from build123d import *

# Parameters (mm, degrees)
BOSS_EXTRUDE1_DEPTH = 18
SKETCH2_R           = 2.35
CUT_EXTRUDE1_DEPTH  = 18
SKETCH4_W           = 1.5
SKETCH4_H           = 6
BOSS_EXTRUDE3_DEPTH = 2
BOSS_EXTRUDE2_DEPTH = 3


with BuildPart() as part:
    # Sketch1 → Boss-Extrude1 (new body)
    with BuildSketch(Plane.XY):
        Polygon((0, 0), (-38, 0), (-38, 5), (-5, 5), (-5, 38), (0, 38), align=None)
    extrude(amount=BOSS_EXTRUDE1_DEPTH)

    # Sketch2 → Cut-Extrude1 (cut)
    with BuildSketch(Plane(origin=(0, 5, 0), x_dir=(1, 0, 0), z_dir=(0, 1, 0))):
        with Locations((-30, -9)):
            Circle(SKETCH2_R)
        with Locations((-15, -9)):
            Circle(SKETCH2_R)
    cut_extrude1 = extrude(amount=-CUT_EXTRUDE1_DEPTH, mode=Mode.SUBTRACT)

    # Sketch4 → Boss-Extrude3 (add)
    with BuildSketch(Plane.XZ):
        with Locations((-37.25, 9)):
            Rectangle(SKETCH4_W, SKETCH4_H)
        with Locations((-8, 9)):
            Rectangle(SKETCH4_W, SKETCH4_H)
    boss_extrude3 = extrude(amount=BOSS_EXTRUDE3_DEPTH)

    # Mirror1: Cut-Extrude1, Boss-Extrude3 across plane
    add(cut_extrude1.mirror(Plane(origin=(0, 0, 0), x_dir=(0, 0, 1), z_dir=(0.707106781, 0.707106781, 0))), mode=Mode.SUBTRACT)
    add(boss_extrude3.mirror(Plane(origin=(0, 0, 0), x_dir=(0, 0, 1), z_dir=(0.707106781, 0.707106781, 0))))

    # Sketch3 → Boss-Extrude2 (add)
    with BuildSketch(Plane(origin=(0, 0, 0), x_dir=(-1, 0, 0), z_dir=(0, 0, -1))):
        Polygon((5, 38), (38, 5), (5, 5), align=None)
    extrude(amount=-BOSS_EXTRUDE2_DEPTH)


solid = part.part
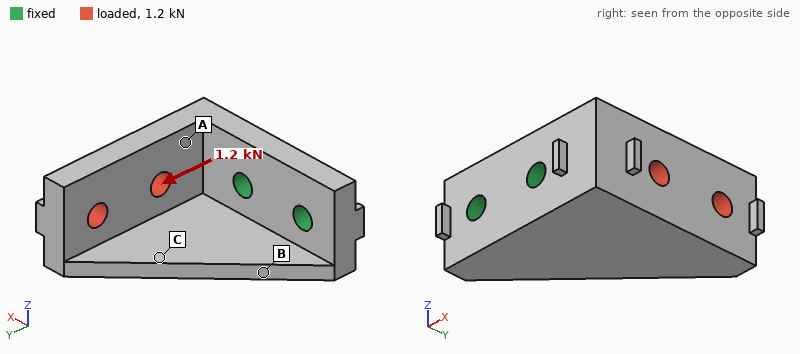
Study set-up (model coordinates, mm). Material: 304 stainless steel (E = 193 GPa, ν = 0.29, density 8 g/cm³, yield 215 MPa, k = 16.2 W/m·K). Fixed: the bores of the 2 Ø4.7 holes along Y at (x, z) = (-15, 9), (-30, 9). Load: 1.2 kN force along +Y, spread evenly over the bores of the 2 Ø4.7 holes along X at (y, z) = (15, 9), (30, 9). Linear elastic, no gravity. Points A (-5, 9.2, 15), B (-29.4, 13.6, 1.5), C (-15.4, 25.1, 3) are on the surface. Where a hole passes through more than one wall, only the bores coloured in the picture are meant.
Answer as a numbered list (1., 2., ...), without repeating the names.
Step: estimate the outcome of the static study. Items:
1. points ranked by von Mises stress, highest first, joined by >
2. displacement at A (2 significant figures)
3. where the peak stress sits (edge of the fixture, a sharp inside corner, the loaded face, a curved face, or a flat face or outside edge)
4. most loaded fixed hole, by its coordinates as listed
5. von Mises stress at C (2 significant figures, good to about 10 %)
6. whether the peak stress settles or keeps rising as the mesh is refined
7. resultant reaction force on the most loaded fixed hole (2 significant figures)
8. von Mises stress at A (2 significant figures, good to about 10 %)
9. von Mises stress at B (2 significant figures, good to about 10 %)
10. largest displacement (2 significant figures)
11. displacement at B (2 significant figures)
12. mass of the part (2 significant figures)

1. A > B > C
2. 11 µm
3. edge of the fixture
4. (-15, 9)
5. 11 MPa
6. keeps rising
7. 1.7 kN
8. 33 MPa
9. 26 MPa
10. 26 µm
11. 4.5 µm
12. 62 g
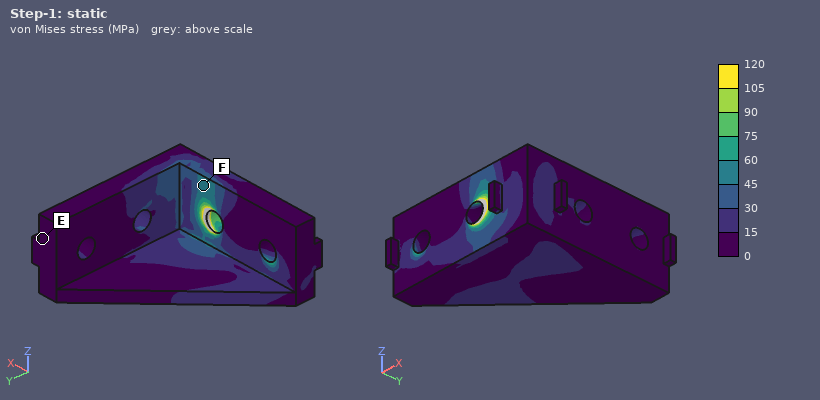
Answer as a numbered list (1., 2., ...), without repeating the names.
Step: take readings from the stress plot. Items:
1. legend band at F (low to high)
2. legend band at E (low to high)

1. 45 to 60 MPa
2. 0 to 15 MPa
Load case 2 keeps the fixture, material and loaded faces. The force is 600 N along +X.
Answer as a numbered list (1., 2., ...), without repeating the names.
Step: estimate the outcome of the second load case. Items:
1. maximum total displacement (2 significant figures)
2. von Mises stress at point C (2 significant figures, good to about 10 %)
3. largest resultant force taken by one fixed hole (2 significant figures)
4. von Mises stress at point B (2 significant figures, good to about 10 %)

1. 43 µm
2. 33 MPa
3. 620 N
4. 30 MPa
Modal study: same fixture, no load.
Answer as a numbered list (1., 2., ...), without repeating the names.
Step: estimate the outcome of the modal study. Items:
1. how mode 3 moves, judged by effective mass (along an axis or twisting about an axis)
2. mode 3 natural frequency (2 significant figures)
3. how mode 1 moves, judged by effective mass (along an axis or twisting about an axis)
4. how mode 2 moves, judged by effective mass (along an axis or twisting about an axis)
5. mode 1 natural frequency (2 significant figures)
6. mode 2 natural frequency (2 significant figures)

1. along Y
2. 10 kHz
3. along Z
4. along X
5. 3400 Hz
6. 5300 Hz
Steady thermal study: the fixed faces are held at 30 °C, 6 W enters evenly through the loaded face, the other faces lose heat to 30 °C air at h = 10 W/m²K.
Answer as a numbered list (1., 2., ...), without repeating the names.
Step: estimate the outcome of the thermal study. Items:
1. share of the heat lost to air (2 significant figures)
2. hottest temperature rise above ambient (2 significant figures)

1. 22 %
2. 74 K
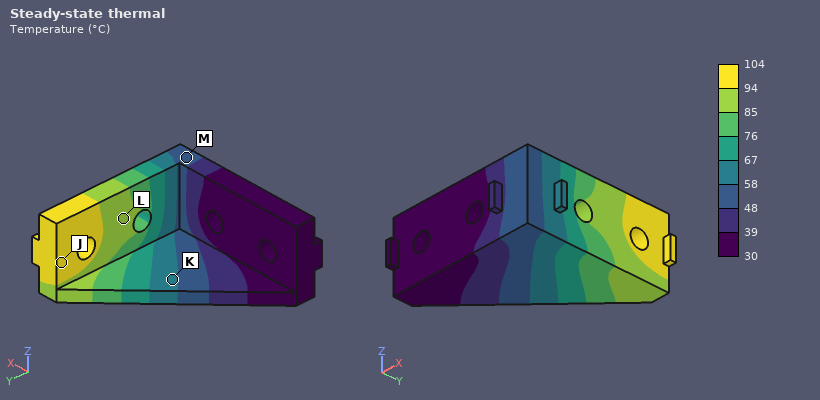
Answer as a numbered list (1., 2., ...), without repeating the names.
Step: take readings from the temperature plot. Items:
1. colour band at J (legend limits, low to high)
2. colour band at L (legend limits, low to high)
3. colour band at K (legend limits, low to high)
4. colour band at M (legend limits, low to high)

1. 94 to 104 °C
2. 85 to 94 °C
3. 58 to 67 °C
4. 48 to 58 °C
